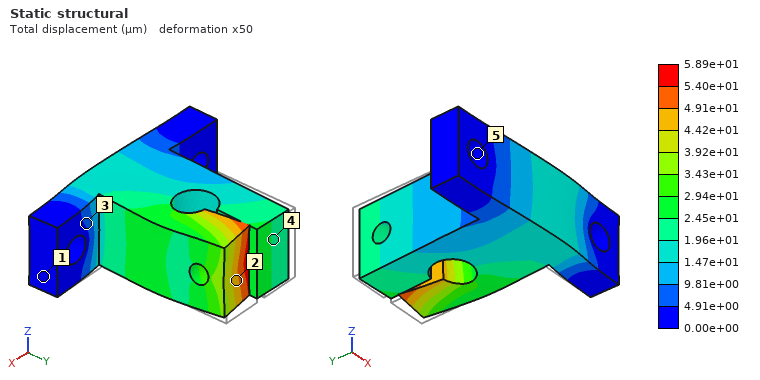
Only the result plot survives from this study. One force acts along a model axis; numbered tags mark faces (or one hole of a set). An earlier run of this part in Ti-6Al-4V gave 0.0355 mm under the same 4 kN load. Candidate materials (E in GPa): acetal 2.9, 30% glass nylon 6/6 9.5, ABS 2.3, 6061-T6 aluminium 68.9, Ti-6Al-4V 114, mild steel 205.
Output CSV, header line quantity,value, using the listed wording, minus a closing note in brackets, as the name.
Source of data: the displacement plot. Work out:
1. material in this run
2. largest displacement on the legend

quantity,value
material in this run,6061-T6 aluminium
largest displacement on the legend,5.89e+01 µm
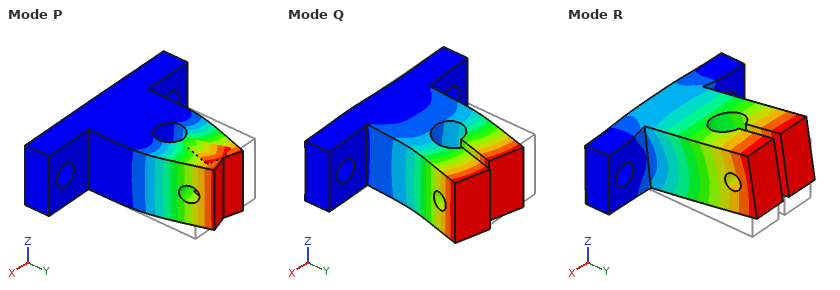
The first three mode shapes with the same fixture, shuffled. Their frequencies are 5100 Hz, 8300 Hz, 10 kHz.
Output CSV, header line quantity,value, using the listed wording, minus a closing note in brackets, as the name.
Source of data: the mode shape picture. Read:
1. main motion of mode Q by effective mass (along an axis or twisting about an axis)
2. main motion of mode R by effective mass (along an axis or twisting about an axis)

quantity,value
main motion of mode Q by effective mass,along X
main motion of mode R by effective mass,along Z
